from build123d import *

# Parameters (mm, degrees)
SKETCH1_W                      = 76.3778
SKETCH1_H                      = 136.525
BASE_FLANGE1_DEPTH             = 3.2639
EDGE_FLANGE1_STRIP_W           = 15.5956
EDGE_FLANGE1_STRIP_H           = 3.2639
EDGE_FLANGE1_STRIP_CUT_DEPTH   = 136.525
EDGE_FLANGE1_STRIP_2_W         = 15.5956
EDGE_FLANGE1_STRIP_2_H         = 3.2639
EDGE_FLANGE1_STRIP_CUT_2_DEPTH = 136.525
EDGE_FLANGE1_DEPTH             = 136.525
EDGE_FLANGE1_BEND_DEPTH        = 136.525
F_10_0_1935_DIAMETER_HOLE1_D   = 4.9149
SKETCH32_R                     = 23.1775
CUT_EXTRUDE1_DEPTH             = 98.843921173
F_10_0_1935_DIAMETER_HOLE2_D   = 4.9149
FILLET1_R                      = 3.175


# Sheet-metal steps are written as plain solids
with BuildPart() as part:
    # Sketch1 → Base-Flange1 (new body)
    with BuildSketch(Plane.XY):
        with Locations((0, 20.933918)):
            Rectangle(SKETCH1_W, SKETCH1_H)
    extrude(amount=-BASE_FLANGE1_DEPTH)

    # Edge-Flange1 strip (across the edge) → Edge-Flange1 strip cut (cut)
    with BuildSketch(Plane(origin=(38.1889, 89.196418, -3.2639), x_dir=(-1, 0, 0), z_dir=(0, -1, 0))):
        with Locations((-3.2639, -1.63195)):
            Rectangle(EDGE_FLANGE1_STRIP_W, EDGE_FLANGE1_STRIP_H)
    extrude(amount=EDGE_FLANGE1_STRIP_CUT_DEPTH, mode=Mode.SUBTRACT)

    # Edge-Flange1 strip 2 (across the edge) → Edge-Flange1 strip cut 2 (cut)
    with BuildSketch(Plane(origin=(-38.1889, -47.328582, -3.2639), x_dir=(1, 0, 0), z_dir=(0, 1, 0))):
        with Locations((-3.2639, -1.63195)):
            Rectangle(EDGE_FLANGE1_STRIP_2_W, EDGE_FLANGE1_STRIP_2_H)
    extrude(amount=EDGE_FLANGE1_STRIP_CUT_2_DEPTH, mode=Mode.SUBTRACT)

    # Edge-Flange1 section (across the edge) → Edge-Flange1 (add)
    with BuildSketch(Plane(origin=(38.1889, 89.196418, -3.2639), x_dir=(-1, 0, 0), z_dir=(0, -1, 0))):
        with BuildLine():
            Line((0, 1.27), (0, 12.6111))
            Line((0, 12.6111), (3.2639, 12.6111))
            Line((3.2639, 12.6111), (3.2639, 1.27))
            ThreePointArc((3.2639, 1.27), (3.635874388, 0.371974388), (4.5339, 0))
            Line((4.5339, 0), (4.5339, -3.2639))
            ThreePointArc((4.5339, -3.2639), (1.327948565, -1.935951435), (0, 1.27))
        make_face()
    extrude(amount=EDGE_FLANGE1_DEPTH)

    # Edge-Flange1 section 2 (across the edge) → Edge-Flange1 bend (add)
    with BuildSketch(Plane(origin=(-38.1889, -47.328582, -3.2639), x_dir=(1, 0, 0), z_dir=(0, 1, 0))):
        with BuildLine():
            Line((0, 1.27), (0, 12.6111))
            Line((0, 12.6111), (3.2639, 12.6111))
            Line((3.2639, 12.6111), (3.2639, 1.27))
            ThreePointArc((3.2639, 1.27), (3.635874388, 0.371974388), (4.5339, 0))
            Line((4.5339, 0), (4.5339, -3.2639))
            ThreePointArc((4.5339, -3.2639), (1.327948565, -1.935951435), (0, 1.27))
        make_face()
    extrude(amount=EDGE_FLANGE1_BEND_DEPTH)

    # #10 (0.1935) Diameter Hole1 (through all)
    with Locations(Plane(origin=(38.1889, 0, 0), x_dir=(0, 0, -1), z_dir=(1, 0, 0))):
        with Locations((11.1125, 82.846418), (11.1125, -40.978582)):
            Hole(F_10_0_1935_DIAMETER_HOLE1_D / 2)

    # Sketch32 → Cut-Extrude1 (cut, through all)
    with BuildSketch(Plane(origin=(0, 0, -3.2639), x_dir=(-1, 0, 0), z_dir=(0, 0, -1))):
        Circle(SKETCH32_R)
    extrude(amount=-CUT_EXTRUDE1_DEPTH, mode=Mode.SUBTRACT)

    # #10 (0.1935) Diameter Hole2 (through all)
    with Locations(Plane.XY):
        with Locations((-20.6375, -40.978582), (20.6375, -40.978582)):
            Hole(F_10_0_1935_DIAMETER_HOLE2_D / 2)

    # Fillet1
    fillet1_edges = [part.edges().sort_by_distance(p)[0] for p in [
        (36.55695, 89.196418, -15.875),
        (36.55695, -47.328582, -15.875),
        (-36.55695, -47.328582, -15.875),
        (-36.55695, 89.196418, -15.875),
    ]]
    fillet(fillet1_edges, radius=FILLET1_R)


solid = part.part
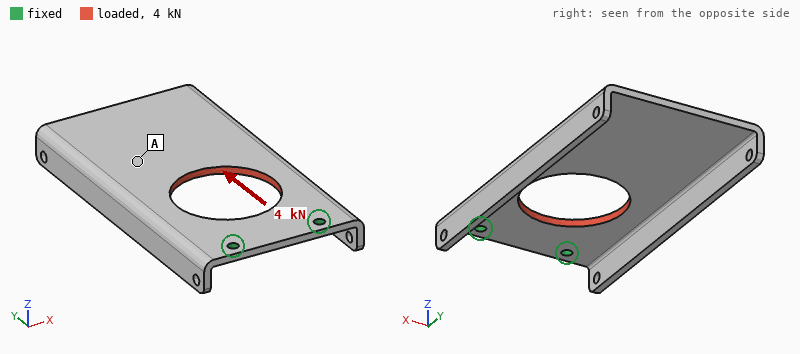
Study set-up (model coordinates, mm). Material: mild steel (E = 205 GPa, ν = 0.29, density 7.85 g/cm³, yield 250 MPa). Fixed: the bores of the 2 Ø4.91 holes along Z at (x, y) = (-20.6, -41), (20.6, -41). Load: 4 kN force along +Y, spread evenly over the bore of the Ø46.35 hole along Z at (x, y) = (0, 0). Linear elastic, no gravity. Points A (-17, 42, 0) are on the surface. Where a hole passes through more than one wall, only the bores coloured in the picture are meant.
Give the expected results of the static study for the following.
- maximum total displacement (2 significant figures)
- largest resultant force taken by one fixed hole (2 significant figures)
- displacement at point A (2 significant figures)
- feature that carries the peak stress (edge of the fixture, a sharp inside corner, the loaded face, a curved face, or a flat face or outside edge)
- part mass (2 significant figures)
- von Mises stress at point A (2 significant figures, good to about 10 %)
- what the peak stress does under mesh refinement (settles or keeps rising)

37 µm
2.0 kN
18 µm
edge of the fixture
300 g
6.2 MPa
keeps rising
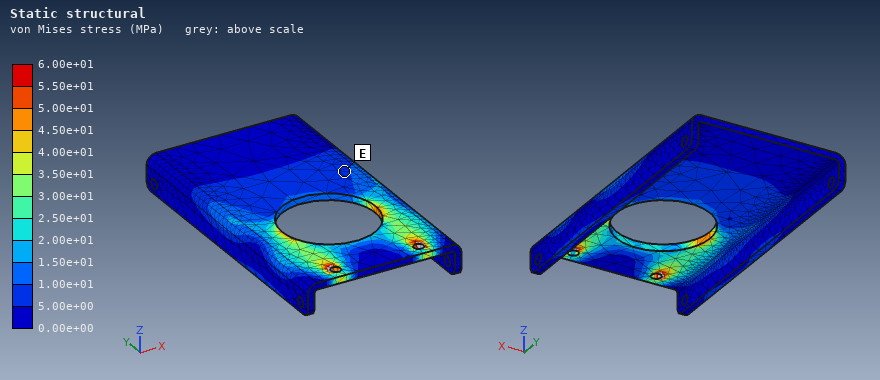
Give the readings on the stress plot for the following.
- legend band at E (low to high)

5.00e+00 to 1.00e+01 MPa
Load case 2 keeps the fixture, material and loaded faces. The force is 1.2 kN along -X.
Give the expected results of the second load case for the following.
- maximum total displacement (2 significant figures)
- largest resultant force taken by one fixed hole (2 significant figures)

35 µm
1.2 kN
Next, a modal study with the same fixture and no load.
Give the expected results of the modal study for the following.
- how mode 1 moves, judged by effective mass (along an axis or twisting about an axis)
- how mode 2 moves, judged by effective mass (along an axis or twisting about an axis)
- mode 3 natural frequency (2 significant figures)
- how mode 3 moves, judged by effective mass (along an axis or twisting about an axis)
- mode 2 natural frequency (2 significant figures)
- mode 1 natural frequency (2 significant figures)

along Z
twisting about Y
1500 Hz
along X
470 Hz
220 Hz
